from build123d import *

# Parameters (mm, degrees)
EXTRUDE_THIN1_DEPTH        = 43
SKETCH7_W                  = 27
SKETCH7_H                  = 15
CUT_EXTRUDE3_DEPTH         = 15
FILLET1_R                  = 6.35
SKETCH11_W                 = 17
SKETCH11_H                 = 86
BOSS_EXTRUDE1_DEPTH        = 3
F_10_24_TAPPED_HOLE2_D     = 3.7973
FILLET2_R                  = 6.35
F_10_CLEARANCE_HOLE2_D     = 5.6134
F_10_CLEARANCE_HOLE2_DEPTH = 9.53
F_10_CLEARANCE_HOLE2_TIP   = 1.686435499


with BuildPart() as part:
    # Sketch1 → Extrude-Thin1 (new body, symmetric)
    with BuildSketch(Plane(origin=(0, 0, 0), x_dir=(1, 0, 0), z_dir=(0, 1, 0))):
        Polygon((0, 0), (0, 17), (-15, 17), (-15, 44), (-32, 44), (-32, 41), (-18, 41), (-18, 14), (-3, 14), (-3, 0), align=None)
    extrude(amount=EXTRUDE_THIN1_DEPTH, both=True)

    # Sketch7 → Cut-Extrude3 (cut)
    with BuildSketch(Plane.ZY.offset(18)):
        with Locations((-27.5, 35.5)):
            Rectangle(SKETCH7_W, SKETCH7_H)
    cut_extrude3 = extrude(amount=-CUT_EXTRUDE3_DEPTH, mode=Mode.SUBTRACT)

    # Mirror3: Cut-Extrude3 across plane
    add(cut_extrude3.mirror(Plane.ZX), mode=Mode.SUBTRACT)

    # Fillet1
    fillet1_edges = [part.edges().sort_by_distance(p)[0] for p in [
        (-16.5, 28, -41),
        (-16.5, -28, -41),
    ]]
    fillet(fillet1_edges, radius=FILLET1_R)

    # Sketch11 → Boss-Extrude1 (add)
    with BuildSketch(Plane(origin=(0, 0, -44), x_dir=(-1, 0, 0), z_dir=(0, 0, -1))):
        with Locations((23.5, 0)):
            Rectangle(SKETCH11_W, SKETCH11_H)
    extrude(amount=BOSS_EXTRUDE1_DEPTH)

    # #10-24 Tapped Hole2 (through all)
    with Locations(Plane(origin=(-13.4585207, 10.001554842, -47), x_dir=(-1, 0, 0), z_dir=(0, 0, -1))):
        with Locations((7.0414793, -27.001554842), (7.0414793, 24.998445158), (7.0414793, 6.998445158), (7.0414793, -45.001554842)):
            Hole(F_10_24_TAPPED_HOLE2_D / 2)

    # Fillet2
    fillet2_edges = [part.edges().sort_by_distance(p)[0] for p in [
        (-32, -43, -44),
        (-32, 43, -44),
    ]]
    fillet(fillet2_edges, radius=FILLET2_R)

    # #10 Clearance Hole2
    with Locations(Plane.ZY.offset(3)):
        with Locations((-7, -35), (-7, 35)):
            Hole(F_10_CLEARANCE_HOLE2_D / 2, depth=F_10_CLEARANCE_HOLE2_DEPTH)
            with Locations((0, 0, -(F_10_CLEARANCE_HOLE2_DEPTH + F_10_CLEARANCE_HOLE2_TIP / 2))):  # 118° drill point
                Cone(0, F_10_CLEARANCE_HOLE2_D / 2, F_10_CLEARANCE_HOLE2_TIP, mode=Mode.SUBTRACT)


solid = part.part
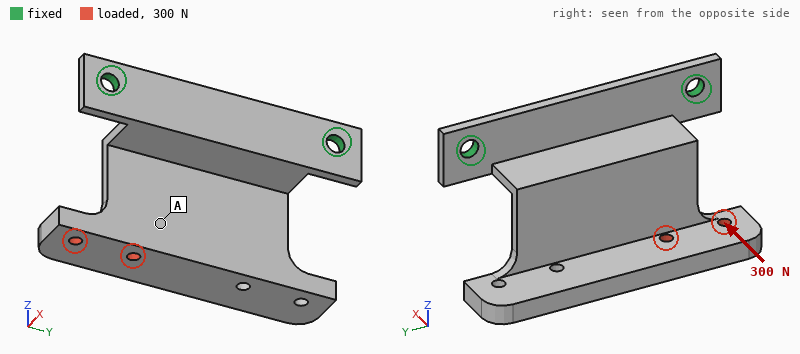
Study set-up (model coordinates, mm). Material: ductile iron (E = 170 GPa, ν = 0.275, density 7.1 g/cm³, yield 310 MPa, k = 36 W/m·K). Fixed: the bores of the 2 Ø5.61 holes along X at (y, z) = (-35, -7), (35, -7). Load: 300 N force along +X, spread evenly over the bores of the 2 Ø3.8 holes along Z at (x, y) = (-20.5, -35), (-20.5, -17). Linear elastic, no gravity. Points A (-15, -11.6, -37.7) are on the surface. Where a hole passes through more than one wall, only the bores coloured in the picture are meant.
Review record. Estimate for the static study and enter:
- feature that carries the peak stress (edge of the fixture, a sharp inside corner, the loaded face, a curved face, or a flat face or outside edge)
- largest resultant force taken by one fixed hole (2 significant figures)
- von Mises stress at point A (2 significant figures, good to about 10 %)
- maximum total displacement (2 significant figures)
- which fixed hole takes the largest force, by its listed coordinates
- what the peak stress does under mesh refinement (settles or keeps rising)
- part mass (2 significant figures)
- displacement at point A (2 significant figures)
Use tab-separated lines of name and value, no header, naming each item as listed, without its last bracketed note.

feature that carries the peak stress	edge of the fixture
largest resultant force taken by one fixed hole	340 N
von Mises stress at point A	30 MPa
maximum total displacement	0.76 mm
which fixed hole takes the largest force, by its listed coordinates	(-35, -7)
what the peak stress does under mesh refinement	keeps rising
part mass	140 g
displacement at point A	0.40 mm
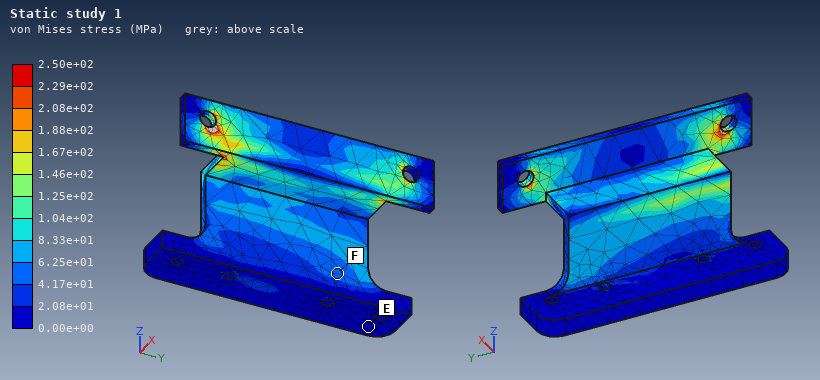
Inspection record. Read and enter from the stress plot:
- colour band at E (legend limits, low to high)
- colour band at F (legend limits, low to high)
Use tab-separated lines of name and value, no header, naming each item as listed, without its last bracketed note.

colour band at E	0.00e+00 to 2.08e+01 MPa
colour band at F	4.17e+01 to 6.25e+01 MPa
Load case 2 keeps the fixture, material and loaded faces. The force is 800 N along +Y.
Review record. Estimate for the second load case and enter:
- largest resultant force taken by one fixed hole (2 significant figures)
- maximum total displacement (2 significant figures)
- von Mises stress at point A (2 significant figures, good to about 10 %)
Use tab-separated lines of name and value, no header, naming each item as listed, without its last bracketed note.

largest resultant force taken by one fixed hole	670 N
maximum total displacement	0.14 mm
von Mises stress at point A	9.7 MPa
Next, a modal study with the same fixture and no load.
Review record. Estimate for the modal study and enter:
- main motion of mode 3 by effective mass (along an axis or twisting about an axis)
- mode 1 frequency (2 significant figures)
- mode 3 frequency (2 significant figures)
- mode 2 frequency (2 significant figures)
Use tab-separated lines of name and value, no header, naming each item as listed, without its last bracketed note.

main motion of mode 3 by effective mass	along Y
mode 1 frequency	430 Hz
mode 3 frequency	1700 Hz
mode 2 frequency	1200 Hz
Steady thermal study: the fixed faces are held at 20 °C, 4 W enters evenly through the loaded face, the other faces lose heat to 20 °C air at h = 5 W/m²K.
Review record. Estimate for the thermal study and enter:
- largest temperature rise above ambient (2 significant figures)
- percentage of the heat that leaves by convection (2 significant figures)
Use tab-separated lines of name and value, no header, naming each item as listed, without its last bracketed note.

largest temperature rise above ambient	48 K
percentage of the heat that leaves by convection	32 %
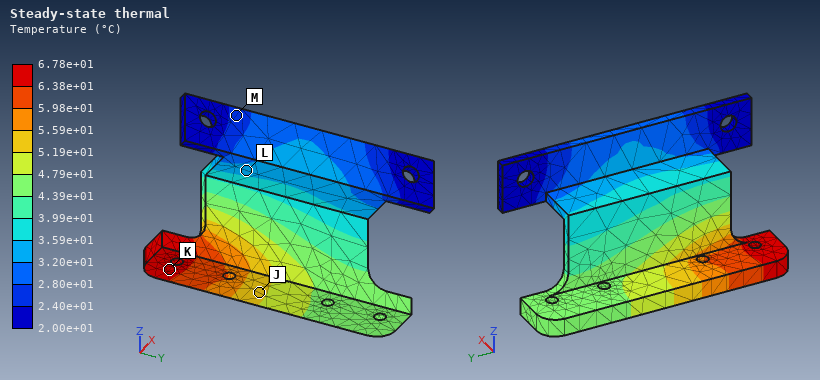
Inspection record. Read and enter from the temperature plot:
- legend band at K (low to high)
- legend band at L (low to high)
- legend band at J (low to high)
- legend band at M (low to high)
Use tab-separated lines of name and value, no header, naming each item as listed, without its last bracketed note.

legend band at K	6.38e+01 to 6.78e+01 °C
legend band at L	3.20e+01 to 3.59e+01 °C
legend band at J	5.19e+01 to 5.59e+01 °C
legend band at M	2.40e+01 to 2.80e+01 °C
